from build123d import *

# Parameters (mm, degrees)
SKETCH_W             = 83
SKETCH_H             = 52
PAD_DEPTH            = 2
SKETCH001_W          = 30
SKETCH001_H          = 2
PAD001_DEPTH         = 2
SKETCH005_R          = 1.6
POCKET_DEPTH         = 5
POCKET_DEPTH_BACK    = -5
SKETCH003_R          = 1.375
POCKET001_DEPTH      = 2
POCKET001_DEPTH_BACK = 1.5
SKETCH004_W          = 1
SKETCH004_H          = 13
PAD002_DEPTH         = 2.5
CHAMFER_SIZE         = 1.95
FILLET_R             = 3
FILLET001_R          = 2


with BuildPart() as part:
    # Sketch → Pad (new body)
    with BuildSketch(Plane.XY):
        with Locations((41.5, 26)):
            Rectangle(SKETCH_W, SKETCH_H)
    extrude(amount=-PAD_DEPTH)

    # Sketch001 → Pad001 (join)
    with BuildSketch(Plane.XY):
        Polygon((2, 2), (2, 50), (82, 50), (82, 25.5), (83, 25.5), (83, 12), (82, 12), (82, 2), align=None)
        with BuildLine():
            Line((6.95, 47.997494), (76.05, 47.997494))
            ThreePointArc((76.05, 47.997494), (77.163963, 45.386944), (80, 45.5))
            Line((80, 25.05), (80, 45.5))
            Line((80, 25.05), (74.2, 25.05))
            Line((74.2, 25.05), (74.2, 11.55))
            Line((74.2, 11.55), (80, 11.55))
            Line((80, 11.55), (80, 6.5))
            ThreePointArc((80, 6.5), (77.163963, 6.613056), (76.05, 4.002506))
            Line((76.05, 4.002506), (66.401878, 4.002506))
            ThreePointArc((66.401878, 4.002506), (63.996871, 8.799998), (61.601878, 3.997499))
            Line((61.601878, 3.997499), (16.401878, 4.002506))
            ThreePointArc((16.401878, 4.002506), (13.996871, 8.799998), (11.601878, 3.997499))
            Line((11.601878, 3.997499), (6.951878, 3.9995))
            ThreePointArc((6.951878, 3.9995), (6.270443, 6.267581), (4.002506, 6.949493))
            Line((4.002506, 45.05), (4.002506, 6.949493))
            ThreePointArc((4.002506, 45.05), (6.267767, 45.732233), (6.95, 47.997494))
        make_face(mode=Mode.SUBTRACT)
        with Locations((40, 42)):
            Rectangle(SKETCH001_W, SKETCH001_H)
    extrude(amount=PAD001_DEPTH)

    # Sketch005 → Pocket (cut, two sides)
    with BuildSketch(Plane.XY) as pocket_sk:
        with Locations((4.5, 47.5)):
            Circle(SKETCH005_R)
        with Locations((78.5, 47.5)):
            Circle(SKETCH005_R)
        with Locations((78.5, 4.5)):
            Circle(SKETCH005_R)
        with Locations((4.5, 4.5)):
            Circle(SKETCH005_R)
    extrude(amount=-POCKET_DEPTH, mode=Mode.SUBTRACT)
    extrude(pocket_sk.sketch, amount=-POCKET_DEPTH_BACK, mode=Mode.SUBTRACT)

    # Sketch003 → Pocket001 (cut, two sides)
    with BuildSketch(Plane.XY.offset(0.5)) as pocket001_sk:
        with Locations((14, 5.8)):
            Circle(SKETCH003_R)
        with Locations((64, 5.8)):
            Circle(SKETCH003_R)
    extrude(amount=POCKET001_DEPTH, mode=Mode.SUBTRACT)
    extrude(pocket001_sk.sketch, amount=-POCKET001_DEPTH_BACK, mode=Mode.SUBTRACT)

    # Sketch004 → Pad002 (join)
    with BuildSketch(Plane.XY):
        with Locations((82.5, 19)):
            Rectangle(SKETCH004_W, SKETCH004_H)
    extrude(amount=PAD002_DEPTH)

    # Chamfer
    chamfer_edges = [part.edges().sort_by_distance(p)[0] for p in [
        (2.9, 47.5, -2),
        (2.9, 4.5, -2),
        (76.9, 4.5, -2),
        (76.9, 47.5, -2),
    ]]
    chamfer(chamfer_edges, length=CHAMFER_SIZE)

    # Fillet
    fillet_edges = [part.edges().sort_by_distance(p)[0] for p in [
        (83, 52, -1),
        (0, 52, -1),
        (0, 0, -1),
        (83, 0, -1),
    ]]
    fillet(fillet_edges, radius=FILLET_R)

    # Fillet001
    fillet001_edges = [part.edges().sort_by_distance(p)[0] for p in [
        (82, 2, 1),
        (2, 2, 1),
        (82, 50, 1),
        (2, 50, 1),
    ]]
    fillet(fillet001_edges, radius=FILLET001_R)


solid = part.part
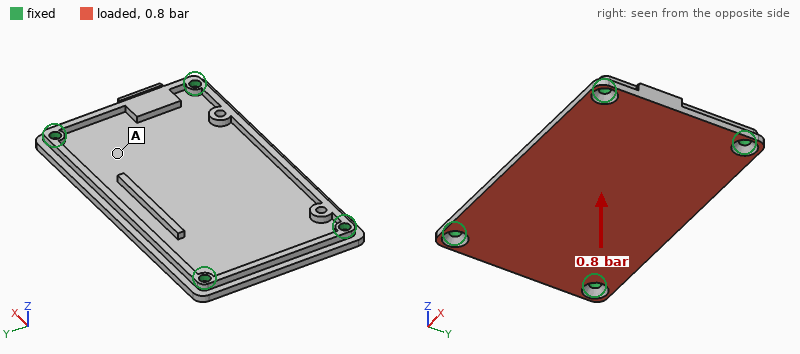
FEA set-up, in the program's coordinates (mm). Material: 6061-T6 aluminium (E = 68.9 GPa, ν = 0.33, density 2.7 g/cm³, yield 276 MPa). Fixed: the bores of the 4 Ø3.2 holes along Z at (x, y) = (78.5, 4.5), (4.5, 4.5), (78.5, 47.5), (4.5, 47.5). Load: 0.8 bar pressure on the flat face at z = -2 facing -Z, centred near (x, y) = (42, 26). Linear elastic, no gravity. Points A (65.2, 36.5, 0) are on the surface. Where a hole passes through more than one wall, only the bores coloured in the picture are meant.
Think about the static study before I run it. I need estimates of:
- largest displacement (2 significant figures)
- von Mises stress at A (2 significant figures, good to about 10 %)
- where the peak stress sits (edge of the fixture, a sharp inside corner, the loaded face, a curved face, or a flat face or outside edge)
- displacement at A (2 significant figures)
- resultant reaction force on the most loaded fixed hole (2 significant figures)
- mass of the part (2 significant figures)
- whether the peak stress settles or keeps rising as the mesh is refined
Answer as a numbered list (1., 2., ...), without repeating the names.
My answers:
1. 0.11 mm
2. 7.4 MPa
3. edge of the fixture
4. 0.054 mm
5. 210 N
6. 26 g
7. keeps rising
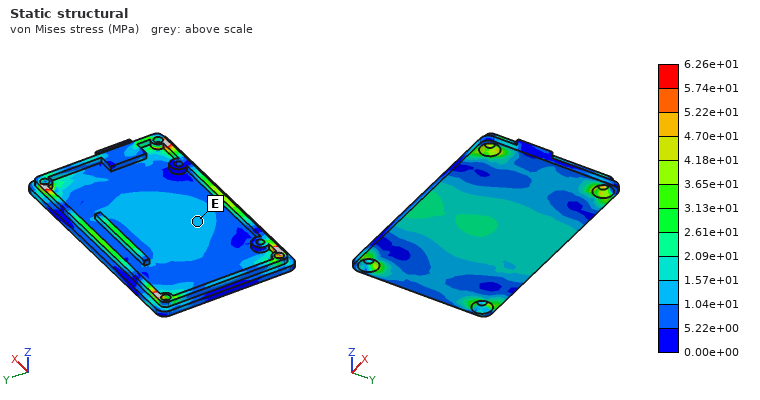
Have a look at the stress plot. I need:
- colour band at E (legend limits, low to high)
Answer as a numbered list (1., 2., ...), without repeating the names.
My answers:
1. 1.04e+01 to 1.57e+01 MPa
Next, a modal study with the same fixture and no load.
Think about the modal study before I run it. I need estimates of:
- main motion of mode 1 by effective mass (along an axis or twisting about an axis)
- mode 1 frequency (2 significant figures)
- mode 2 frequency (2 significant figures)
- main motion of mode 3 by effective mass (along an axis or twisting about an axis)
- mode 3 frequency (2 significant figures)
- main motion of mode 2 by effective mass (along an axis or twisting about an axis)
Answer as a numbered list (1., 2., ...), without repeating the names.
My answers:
1. along Z
2. 2100 Hz
3. 3200 Hz
4. twisting about Y
5. 4900 Hz
6. twisting about X
